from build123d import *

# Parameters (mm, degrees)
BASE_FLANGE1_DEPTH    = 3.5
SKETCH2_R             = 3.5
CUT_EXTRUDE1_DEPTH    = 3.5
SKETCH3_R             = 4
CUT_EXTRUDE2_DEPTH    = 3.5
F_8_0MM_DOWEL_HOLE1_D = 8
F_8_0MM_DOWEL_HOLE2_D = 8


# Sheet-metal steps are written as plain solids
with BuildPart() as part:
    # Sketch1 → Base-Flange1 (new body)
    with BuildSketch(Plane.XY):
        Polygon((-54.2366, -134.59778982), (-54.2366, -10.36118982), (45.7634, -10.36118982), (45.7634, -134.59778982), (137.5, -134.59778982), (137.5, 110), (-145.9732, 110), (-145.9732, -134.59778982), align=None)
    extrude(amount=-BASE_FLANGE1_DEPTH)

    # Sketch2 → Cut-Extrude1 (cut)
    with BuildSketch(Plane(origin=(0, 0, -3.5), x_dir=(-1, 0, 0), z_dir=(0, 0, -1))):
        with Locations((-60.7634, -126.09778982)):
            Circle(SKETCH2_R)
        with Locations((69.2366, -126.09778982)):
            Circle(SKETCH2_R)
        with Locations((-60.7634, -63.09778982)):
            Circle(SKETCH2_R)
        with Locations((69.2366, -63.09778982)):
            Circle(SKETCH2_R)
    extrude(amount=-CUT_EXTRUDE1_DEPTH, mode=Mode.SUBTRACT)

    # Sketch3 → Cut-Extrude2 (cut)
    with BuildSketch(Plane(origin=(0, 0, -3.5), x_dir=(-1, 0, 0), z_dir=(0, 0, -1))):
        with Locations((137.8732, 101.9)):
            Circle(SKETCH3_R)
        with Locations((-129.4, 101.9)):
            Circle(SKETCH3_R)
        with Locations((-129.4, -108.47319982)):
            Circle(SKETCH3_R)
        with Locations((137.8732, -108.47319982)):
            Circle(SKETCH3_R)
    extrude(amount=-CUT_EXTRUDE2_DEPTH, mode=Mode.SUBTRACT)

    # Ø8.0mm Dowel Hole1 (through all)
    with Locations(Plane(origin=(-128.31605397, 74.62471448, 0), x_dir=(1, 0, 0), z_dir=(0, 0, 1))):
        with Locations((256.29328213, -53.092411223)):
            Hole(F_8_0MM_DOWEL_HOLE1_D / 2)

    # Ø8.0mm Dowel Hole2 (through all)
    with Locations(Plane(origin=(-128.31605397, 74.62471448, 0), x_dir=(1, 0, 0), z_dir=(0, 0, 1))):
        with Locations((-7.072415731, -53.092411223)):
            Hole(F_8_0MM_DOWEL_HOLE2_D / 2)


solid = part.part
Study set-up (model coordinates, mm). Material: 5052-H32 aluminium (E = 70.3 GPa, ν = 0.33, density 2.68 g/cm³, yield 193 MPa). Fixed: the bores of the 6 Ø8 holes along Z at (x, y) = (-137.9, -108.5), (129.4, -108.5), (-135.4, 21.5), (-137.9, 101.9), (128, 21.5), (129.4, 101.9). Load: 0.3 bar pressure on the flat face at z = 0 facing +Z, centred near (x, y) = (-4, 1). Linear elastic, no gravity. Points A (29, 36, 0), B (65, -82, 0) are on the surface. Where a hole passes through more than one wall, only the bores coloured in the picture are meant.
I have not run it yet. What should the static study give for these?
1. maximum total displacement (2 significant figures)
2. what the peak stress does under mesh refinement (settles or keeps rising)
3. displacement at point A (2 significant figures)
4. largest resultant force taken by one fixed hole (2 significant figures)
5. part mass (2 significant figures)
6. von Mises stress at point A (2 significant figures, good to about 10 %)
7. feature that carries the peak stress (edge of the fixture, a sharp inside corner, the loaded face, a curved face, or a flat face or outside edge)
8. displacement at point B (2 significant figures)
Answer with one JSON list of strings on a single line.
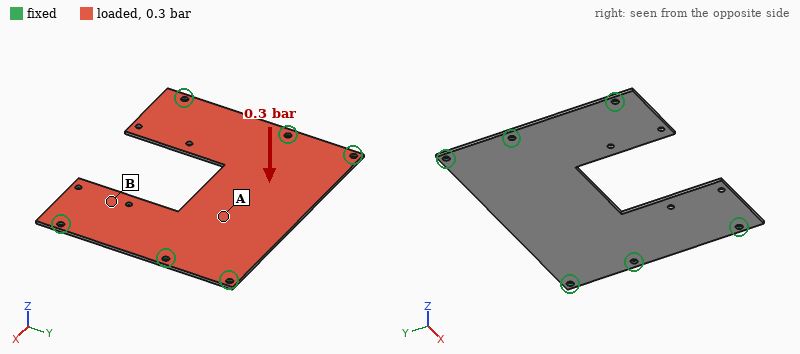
["1.8 mm", "keeps rising", "1.5 mm", "430 N", "530 g", "35 MPa", "edge of the fixture", "0.93 mm"]
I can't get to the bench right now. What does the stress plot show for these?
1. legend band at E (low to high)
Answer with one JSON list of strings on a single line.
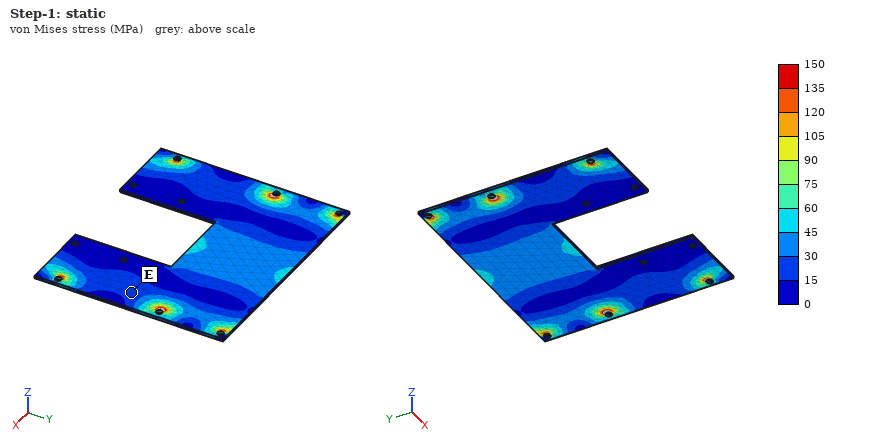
["15 to 30 MPa"]
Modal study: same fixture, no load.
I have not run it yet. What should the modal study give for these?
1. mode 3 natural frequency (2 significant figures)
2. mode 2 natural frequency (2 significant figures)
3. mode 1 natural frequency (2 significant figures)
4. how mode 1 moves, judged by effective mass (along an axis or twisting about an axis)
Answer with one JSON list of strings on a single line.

["460 Hz", "390 Hz", "260 Hz", "along Z"]
